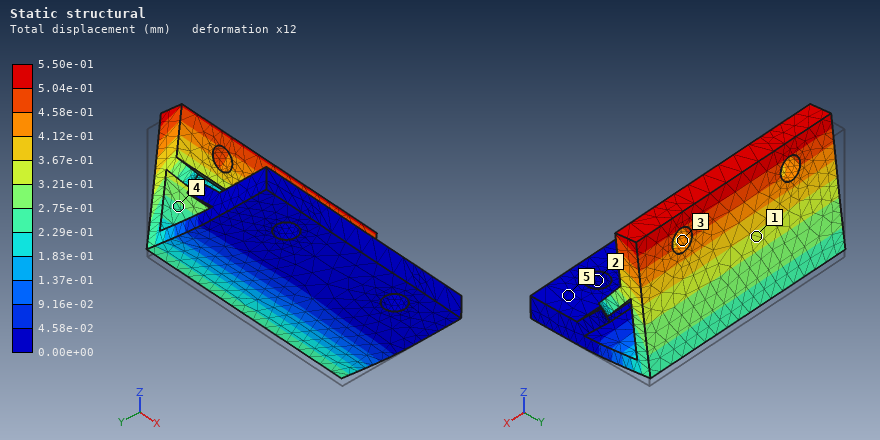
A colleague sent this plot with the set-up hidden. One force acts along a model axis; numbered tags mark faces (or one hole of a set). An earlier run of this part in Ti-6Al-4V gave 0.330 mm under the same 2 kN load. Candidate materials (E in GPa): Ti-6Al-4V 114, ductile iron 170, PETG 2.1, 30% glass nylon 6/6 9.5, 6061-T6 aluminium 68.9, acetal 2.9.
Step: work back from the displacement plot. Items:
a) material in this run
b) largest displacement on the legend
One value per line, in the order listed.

6061-T6 aluminium
5.50e-01 mm
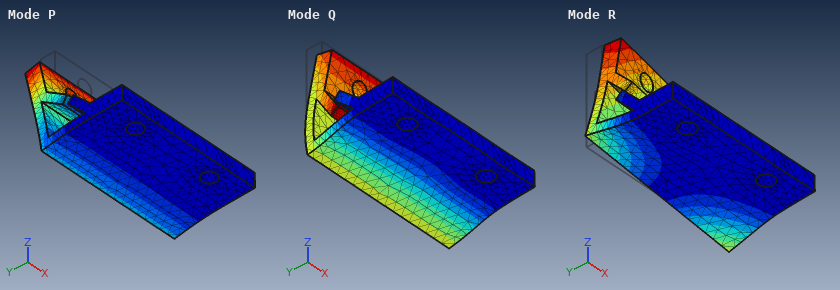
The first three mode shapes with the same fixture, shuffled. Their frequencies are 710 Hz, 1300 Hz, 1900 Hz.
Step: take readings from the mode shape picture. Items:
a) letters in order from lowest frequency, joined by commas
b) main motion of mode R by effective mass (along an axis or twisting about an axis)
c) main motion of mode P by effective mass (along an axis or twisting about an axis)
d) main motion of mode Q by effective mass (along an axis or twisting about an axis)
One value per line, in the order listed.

P, R, Q
along X
along Y
along Z
